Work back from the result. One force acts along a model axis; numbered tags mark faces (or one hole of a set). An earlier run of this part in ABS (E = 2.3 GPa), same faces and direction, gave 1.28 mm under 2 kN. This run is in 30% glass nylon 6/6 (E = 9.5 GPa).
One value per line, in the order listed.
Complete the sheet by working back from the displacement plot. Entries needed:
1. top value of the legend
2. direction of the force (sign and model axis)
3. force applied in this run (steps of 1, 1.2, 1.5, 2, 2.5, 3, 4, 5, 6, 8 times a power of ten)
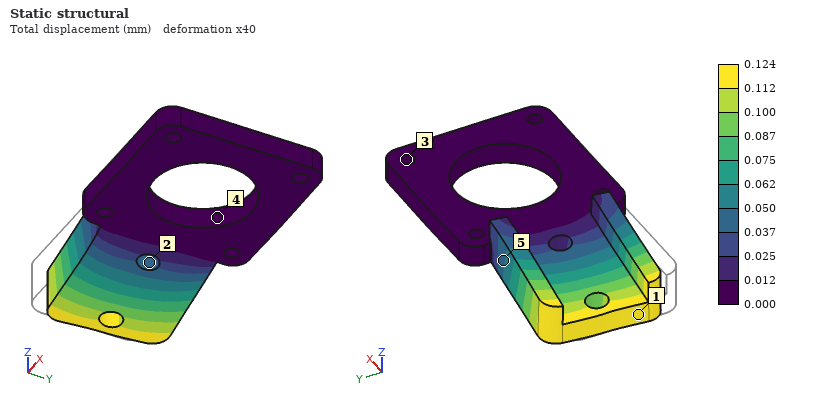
0.124 mm
+Y
800 N
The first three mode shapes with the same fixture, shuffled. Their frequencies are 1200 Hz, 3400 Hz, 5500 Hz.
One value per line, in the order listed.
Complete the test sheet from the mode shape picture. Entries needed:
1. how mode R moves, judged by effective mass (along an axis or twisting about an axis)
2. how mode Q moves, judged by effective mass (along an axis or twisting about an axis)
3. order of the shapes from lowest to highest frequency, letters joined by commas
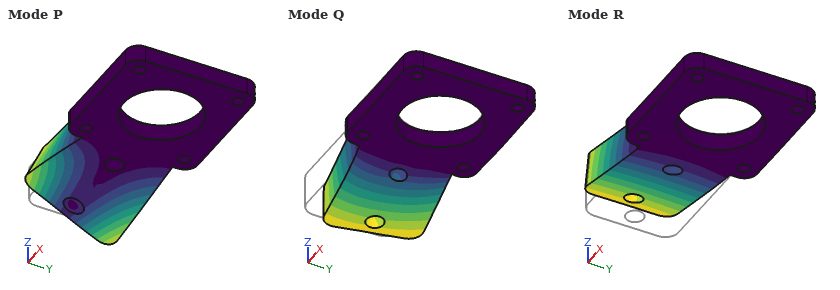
along Z
along Y
R, P, Q
